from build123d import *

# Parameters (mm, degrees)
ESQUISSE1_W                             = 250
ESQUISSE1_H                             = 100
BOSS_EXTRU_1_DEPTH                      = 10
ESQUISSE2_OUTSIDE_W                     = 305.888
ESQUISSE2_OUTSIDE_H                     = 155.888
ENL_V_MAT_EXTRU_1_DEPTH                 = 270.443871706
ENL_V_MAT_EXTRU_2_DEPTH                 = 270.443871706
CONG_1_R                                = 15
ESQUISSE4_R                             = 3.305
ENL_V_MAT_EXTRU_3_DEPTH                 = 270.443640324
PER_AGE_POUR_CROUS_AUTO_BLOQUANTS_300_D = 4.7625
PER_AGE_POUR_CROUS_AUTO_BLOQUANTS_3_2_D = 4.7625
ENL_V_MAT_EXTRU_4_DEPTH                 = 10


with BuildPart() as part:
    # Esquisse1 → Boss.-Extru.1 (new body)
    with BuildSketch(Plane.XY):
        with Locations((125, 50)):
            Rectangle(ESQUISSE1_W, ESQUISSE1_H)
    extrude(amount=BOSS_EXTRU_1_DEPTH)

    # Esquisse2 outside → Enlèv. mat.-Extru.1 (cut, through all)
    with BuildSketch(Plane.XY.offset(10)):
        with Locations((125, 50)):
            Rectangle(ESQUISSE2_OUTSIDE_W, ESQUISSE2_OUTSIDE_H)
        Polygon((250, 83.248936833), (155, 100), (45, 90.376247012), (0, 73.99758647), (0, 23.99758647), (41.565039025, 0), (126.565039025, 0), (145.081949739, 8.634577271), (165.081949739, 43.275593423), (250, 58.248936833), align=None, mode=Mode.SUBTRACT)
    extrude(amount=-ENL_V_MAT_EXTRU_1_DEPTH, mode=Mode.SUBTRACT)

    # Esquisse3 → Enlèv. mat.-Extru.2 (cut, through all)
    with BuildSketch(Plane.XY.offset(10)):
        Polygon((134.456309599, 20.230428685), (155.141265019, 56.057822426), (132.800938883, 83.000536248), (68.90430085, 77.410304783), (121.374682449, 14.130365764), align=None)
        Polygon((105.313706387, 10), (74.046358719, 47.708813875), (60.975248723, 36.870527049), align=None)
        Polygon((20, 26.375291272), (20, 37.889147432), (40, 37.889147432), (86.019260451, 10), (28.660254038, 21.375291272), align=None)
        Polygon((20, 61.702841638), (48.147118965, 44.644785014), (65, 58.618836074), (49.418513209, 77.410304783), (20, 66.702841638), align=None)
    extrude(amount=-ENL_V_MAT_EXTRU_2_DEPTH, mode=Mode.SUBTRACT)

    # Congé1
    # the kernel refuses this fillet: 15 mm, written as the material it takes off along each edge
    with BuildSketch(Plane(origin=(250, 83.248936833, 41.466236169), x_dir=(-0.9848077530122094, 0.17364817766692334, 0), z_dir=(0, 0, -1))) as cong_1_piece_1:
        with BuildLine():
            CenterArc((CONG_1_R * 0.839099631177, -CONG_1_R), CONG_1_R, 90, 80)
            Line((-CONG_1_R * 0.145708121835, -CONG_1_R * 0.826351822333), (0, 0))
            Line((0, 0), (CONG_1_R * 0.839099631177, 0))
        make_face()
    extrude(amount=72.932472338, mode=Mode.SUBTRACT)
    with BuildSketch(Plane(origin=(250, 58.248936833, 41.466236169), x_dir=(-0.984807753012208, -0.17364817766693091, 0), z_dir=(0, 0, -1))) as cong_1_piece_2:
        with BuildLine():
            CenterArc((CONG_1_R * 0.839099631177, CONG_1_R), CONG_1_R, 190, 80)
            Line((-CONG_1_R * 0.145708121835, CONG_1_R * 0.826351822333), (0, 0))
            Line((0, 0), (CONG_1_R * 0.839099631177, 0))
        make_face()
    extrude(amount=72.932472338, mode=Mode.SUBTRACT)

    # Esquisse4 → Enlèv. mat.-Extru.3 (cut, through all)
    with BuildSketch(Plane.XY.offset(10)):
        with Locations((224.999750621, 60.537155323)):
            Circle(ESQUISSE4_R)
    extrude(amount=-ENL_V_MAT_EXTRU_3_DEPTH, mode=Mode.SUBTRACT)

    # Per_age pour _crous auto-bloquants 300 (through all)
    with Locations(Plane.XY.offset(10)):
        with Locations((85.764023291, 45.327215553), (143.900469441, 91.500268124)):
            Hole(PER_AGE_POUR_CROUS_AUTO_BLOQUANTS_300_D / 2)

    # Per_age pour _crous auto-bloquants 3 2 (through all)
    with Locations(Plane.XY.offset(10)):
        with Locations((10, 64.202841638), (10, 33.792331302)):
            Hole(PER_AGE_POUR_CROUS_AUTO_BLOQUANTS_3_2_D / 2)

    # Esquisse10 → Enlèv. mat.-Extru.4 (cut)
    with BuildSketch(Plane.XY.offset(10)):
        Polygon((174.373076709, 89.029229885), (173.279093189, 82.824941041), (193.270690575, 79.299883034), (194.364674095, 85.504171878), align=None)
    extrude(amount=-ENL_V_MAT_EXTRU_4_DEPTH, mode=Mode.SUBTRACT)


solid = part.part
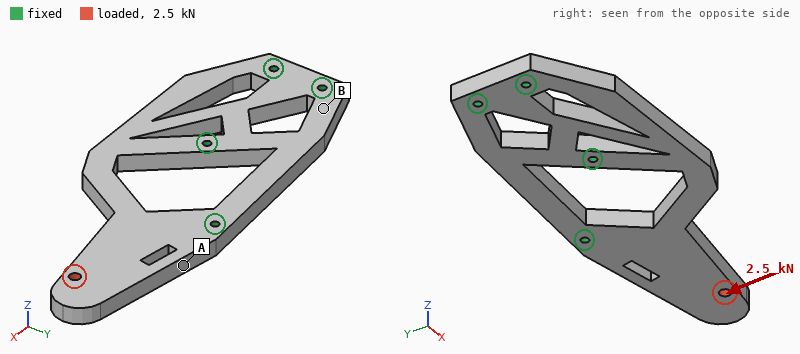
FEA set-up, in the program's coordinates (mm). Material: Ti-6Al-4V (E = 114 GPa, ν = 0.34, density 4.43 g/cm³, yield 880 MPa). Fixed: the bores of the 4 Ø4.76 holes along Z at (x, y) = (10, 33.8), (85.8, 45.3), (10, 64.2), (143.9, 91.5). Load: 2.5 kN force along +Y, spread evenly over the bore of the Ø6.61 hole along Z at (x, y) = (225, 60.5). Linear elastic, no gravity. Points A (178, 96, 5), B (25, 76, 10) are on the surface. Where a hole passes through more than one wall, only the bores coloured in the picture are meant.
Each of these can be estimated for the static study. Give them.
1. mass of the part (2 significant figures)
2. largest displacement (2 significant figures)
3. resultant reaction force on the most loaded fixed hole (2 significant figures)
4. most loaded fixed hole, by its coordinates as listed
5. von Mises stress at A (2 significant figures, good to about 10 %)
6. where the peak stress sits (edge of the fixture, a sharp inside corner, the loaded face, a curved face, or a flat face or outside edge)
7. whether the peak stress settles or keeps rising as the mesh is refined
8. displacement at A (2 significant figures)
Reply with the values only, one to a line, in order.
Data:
530 g
0.19 mm
2.9 kN
(143.9, 91.5)
33 MPa
edge of the fixture
keeps rising
0.052 mm
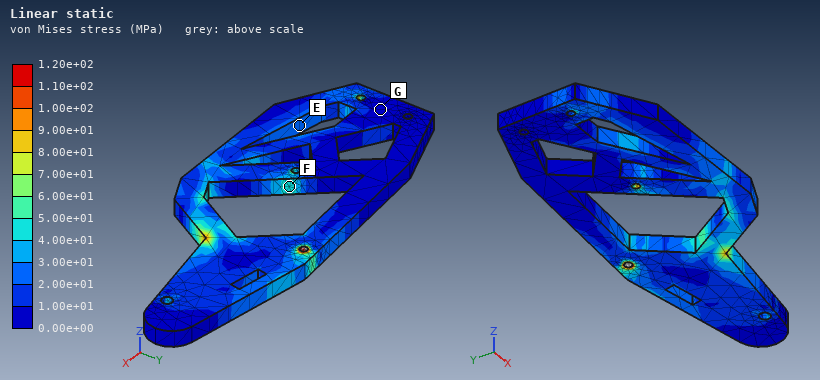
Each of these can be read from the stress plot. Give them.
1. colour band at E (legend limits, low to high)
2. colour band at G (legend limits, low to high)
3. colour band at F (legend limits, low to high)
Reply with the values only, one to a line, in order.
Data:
2.00e+01 to 3.00e+01 MPa
0.00e+00 to 1.00e+01 MPa
4.00e+01 to 5.00e+01 MPa
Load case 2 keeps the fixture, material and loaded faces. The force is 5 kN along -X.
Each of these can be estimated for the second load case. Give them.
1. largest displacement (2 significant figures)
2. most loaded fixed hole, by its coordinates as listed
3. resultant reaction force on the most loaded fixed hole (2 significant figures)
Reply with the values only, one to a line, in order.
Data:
0.13 mm
(143.9, 91.5)
3.1 kN
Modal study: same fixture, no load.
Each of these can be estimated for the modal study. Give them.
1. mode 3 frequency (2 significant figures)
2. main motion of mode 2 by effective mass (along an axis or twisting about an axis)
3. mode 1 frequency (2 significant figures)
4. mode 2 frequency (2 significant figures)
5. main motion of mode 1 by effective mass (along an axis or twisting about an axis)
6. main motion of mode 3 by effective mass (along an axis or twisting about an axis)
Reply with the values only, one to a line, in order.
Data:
2100 Hz
along Z
720 Hz
1700 Hz
along Z
along Y
